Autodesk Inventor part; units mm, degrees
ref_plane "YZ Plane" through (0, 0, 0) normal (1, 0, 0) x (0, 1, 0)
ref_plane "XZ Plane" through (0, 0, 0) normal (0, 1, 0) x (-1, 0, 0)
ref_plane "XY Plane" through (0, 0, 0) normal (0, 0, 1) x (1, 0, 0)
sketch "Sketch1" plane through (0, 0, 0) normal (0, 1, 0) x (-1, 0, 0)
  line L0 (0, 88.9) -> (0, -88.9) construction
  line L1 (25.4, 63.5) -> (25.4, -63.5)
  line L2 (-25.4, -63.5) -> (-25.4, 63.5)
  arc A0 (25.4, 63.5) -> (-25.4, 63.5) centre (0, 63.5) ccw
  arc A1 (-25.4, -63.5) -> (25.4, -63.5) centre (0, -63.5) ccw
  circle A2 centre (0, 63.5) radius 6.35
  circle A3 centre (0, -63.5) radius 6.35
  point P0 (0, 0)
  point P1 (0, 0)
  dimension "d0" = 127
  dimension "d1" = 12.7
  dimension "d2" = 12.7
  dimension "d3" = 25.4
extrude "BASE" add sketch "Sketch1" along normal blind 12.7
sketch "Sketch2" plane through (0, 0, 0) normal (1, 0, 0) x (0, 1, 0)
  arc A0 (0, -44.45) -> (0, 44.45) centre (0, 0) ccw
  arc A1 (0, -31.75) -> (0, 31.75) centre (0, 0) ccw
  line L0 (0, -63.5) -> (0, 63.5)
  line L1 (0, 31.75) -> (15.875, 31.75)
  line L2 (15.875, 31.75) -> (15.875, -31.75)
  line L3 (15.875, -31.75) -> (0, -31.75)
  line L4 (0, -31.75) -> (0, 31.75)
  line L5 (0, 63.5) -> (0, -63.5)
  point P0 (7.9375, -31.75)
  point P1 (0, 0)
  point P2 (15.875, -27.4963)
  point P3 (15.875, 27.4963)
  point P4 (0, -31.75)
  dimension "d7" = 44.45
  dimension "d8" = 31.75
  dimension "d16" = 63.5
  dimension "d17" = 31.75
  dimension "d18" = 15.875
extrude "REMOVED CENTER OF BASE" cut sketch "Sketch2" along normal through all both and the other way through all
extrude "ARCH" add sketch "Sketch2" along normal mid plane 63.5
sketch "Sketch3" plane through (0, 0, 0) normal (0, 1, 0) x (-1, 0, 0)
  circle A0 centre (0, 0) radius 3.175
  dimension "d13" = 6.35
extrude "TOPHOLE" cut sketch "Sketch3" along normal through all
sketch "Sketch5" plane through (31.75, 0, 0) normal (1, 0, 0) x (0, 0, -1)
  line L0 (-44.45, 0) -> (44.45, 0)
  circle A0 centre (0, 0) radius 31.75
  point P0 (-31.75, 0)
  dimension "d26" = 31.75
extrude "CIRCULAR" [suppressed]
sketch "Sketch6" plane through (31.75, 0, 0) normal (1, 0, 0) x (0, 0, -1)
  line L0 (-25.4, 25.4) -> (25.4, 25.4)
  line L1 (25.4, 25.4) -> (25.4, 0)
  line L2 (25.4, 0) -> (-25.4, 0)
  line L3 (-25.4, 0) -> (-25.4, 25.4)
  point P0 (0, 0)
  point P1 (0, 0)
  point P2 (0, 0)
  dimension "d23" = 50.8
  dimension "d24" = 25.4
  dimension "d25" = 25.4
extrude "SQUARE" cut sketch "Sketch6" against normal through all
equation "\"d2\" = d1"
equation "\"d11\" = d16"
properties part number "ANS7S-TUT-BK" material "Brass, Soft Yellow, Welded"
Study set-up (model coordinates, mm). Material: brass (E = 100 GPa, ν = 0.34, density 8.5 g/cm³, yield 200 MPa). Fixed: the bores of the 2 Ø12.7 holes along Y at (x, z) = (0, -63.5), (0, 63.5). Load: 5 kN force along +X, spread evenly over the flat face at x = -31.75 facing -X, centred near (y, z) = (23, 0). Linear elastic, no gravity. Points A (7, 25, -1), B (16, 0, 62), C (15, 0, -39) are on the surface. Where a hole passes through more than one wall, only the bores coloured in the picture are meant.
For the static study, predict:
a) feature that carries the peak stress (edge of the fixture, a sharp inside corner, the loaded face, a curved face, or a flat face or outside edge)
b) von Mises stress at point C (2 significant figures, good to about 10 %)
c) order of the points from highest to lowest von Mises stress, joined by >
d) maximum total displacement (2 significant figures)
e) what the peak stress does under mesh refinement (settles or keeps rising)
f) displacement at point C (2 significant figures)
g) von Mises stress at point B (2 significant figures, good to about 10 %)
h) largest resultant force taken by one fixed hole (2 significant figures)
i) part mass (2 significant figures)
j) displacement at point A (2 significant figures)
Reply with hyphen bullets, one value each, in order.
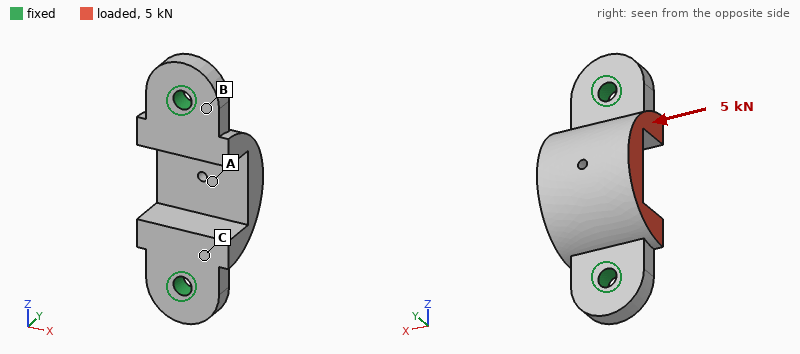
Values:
- edge of the fixture
- 9.2 MPa
- B > C > A
- 52 µm
- keeps rising
- 12 µm
- 19 MPa
- 2.5 kN
- 1.4 kg
- 27 µm
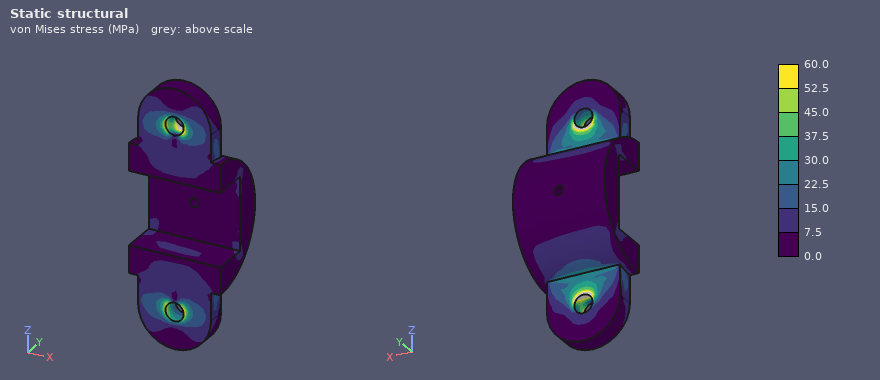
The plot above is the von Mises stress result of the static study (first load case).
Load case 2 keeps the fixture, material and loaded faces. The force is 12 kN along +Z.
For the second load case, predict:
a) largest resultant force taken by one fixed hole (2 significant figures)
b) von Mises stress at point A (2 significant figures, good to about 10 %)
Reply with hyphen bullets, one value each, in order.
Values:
- 6.7 kN
- 20 MPa
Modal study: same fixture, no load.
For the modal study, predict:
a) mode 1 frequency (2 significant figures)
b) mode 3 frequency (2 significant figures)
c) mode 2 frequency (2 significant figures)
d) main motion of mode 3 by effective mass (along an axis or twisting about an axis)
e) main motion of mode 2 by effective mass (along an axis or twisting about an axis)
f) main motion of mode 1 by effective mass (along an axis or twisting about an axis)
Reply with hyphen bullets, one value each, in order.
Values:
- 1800 Hz
- 3800 Hz
- 3600 Hz
- along Z
- along Y
- along X
